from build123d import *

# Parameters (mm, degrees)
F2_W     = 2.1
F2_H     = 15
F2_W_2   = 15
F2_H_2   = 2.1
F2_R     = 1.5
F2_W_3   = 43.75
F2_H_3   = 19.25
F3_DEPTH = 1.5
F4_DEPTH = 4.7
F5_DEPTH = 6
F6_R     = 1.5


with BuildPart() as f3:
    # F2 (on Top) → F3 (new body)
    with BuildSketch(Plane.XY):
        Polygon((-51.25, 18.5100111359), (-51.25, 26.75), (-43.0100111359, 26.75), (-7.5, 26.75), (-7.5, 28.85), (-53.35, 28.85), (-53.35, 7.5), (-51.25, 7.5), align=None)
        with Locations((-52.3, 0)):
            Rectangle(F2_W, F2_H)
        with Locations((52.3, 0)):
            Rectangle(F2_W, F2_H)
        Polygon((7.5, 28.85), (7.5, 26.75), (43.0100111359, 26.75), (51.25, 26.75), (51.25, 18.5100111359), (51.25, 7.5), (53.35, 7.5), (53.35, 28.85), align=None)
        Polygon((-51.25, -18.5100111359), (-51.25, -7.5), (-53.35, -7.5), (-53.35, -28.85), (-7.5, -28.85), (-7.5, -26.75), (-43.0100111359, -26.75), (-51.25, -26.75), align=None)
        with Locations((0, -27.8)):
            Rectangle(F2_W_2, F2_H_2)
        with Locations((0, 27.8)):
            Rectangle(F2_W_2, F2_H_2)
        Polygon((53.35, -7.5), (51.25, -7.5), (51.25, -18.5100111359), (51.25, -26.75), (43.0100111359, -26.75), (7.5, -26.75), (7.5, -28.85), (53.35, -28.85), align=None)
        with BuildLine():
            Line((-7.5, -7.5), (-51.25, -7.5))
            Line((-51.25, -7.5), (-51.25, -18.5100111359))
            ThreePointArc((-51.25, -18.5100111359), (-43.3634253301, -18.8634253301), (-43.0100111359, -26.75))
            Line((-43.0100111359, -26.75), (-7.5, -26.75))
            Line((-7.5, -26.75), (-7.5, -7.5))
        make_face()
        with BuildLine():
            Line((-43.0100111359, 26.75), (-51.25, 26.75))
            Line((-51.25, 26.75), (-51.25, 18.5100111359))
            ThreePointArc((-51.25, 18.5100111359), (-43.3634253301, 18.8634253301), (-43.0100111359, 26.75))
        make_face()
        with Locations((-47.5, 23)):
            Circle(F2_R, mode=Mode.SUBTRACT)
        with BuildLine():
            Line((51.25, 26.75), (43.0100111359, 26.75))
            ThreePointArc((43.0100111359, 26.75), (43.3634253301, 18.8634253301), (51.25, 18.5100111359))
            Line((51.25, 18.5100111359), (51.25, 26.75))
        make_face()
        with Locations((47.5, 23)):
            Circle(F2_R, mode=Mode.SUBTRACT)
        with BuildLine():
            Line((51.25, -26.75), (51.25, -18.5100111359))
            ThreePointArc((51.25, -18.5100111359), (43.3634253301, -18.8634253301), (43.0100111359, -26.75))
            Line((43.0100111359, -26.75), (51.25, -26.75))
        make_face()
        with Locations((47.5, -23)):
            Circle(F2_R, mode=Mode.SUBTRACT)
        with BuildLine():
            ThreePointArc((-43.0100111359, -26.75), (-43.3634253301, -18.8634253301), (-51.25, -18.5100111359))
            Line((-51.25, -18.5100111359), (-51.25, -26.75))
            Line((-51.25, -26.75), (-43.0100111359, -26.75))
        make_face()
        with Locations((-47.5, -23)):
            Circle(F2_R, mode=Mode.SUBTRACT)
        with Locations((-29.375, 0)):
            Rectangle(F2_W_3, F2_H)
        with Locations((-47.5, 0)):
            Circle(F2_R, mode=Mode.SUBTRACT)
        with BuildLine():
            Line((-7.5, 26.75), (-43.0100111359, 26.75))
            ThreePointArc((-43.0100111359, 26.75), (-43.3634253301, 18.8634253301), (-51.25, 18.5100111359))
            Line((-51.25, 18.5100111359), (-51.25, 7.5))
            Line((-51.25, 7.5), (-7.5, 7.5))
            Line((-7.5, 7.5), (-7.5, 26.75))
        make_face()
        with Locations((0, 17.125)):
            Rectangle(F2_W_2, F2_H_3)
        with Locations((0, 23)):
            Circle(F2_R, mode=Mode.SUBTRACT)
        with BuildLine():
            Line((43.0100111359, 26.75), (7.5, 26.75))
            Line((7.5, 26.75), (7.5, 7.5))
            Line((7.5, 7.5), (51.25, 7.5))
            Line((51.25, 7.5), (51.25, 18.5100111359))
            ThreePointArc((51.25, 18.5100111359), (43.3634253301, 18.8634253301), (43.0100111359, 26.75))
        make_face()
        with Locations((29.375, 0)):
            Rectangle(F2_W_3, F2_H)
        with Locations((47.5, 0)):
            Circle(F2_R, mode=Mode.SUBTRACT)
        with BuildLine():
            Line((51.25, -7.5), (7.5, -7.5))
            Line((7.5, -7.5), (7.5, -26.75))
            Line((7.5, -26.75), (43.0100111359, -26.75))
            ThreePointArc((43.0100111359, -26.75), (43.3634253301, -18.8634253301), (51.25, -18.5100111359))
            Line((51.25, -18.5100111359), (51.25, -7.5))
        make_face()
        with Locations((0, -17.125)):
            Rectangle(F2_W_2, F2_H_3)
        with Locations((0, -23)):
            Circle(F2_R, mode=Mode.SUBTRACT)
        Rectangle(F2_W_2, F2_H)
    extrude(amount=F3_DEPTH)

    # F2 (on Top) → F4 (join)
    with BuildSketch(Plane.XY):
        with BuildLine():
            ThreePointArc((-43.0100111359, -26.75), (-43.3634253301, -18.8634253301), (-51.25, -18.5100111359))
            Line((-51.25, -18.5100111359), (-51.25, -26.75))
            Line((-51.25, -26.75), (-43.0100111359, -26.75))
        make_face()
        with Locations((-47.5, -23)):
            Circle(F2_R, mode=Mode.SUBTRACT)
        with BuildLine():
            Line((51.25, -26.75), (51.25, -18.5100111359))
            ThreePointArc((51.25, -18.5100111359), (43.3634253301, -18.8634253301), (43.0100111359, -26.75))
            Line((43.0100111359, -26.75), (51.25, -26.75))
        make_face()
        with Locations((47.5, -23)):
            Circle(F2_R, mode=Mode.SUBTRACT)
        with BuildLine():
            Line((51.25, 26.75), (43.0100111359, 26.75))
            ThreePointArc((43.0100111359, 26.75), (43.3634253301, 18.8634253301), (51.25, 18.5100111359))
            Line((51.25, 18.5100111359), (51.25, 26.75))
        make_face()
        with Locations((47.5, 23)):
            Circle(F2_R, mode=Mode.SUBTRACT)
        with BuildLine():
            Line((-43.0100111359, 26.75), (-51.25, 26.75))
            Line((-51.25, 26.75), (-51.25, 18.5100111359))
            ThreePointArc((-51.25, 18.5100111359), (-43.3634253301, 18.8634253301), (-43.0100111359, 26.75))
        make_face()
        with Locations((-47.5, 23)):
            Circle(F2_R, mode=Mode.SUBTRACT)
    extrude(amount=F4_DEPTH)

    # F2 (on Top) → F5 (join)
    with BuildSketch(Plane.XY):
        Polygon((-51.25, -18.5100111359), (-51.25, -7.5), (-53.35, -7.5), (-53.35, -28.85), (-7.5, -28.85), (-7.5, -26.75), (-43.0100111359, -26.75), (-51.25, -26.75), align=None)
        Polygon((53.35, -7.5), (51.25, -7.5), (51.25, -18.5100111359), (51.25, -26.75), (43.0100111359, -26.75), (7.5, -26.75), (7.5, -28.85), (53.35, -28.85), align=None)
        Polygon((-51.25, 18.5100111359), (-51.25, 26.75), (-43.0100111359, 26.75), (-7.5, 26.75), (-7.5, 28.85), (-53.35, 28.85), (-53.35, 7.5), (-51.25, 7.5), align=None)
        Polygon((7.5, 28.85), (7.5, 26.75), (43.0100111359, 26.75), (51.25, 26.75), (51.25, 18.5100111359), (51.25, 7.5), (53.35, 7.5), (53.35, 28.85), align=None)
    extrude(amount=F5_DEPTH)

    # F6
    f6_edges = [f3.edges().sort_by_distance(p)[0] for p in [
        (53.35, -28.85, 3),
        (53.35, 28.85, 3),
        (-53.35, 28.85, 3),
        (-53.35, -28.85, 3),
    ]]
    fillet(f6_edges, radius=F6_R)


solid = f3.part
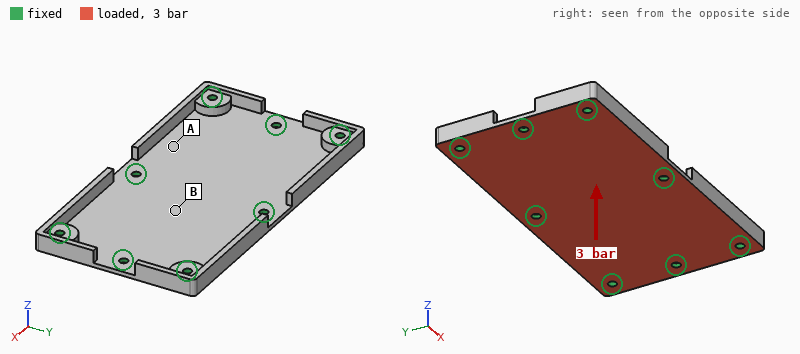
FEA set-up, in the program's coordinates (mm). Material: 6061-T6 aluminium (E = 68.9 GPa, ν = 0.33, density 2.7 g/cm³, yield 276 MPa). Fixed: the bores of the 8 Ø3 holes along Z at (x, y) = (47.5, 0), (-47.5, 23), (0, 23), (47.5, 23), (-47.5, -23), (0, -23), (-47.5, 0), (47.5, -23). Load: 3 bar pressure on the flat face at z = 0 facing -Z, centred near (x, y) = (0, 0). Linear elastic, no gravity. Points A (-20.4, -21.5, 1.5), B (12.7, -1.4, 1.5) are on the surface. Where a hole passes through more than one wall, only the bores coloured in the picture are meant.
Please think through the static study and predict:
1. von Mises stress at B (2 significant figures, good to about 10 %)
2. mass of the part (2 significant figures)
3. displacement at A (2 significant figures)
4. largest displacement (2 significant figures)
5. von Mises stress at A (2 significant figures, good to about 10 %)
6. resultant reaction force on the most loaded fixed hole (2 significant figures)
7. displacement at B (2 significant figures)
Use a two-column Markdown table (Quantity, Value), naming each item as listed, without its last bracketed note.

| Quantity | Value |
|---|---|
| von Mises stress at B | 68 MPa |
| mass of the part | 34 g |
| displacement at A | 0.084 mm |
| largest displacement | 0.26 mm |
| von Mises stress at A | 22 MPa |
| resultant reaction force on the most loaded fixed hole | 370 N |
| displacement at B | 0.26 mm |
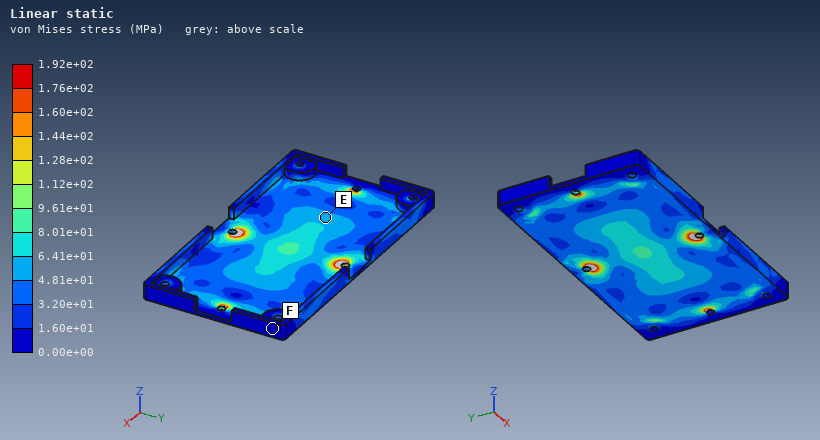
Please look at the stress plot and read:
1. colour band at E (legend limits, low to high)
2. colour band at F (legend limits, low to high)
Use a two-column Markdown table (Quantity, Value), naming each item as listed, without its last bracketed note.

| Quantity | Value |
|---|---|
| colour band at E | 4.81e+01 to 6.41e+01 MPa |
| colour band at F | 0.00e+00 to 1.60e+01 MPa |
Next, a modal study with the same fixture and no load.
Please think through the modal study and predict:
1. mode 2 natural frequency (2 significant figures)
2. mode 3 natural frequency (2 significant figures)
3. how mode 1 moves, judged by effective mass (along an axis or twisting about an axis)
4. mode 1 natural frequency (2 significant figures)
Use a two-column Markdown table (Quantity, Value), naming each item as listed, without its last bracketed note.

| Quantity | Value |
|---|---|
| mode 2 natural frequency | 3800 Hz |
| mode 3 natural frequency | 6500 Hz |
| how mode 1 moves, judged by effective mass | along Z |
| mode 1 natural frequency | 3200 Hz |
